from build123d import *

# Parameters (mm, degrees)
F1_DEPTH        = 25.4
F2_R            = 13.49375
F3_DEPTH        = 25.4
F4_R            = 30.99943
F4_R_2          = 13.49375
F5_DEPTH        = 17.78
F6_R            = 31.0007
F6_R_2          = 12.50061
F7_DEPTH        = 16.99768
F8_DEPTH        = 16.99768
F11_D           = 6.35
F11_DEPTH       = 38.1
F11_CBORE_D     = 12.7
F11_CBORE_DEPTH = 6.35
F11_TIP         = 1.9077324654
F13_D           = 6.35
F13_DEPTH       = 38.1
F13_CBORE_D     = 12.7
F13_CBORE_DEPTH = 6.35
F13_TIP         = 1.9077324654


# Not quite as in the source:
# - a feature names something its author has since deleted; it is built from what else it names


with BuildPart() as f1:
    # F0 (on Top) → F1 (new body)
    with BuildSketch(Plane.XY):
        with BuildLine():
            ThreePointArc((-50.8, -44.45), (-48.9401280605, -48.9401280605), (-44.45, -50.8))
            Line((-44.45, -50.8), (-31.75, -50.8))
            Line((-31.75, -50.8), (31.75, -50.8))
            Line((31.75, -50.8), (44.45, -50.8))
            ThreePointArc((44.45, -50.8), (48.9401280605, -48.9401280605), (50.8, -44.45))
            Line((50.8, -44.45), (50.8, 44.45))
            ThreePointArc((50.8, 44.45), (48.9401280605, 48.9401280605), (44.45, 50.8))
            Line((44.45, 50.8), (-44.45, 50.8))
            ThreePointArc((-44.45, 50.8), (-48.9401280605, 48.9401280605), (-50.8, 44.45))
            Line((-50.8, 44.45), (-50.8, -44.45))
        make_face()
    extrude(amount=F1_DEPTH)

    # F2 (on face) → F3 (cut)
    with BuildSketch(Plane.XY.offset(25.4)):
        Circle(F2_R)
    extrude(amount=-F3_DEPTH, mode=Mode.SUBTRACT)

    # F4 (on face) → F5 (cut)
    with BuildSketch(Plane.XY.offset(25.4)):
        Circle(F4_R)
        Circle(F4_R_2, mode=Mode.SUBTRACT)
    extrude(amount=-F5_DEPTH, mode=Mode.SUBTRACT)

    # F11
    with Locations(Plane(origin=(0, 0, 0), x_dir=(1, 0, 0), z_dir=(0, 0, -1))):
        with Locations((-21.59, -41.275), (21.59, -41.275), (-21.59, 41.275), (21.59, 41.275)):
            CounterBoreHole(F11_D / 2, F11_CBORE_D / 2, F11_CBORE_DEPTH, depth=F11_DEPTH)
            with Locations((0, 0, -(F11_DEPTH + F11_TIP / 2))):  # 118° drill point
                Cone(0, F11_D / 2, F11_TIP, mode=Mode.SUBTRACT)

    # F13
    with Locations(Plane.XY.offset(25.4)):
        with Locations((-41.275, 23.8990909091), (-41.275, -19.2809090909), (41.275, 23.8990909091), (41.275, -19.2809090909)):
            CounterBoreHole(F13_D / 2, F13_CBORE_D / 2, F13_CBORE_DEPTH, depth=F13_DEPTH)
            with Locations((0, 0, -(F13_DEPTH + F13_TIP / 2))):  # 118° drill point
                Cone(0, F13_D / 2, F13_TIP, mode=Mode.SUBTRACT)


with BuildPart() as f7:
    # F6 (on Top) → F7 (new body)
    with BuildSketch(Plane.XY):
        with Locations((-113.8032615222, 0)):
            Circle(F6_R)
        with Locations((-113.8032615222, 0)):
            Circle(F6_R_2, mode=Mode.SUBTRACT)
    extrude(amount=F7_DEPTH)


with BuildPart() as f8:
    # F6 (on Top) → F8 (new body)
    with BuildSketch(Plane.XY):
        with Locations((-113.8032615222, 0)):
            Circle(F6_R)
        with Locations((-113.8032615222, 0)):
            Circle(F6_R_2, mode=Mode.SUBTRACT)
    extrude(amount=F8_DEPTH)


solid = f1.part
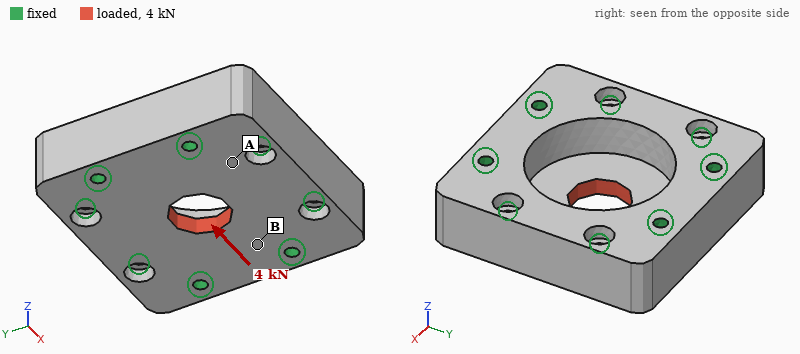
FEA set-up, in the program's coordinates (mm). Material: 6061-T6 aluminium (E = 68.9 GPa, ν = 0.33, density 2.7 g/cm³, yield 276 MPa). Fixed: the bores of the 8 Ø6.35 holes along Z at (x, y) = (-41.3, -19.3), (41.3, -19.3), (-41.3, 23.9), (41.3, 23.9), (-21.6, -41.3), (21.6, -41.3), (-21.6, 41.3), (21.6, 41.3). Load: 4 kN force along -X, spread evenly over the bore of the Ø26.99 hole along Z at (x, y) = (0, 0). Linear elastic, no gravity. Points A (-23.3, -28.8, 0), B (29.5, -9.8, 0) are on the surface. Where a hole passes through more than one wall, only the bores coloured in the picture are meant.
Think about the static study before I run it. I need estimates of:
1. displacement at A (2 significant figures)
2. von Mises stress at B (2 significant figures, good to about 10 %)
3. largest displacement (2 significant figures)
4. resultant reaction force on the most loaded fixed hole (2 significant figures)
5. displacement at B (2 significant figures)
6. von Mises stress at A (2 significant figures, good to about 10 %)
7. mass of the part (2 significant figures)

0.60 µm
4.3 MPa
2.7 µm
860 N
1.3 µm
2.0 MPa
520 g
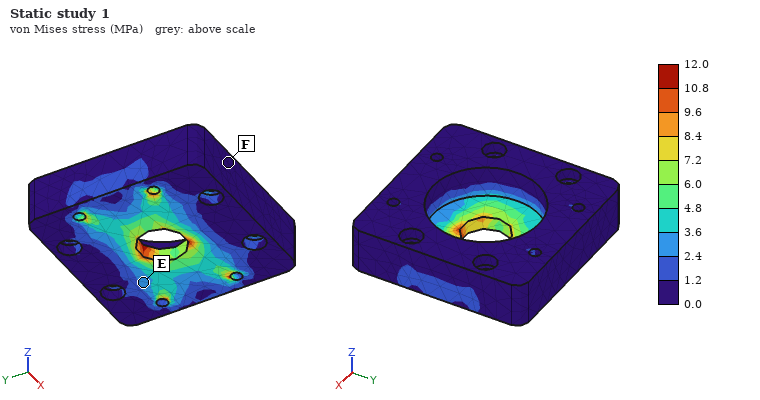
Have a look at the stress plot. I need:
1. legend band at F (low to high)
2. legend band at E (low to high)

0.0 to 1.2 MPa
2.4 to 3.6 MPa
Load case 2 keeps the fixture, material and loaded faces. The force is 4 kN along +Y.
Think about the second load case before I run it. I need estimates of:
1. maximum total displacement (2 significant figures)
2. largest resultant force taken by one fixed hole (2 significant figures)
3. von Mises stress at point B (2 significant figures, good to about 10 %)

3.2 µm
690 N
2.1 MPa
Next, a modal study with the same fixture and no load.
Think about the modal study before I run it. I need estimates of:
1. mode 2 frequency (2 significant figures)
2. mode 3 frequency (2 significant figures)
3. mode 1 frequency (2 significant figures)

19 kHz
20 kHz
15 kHz
